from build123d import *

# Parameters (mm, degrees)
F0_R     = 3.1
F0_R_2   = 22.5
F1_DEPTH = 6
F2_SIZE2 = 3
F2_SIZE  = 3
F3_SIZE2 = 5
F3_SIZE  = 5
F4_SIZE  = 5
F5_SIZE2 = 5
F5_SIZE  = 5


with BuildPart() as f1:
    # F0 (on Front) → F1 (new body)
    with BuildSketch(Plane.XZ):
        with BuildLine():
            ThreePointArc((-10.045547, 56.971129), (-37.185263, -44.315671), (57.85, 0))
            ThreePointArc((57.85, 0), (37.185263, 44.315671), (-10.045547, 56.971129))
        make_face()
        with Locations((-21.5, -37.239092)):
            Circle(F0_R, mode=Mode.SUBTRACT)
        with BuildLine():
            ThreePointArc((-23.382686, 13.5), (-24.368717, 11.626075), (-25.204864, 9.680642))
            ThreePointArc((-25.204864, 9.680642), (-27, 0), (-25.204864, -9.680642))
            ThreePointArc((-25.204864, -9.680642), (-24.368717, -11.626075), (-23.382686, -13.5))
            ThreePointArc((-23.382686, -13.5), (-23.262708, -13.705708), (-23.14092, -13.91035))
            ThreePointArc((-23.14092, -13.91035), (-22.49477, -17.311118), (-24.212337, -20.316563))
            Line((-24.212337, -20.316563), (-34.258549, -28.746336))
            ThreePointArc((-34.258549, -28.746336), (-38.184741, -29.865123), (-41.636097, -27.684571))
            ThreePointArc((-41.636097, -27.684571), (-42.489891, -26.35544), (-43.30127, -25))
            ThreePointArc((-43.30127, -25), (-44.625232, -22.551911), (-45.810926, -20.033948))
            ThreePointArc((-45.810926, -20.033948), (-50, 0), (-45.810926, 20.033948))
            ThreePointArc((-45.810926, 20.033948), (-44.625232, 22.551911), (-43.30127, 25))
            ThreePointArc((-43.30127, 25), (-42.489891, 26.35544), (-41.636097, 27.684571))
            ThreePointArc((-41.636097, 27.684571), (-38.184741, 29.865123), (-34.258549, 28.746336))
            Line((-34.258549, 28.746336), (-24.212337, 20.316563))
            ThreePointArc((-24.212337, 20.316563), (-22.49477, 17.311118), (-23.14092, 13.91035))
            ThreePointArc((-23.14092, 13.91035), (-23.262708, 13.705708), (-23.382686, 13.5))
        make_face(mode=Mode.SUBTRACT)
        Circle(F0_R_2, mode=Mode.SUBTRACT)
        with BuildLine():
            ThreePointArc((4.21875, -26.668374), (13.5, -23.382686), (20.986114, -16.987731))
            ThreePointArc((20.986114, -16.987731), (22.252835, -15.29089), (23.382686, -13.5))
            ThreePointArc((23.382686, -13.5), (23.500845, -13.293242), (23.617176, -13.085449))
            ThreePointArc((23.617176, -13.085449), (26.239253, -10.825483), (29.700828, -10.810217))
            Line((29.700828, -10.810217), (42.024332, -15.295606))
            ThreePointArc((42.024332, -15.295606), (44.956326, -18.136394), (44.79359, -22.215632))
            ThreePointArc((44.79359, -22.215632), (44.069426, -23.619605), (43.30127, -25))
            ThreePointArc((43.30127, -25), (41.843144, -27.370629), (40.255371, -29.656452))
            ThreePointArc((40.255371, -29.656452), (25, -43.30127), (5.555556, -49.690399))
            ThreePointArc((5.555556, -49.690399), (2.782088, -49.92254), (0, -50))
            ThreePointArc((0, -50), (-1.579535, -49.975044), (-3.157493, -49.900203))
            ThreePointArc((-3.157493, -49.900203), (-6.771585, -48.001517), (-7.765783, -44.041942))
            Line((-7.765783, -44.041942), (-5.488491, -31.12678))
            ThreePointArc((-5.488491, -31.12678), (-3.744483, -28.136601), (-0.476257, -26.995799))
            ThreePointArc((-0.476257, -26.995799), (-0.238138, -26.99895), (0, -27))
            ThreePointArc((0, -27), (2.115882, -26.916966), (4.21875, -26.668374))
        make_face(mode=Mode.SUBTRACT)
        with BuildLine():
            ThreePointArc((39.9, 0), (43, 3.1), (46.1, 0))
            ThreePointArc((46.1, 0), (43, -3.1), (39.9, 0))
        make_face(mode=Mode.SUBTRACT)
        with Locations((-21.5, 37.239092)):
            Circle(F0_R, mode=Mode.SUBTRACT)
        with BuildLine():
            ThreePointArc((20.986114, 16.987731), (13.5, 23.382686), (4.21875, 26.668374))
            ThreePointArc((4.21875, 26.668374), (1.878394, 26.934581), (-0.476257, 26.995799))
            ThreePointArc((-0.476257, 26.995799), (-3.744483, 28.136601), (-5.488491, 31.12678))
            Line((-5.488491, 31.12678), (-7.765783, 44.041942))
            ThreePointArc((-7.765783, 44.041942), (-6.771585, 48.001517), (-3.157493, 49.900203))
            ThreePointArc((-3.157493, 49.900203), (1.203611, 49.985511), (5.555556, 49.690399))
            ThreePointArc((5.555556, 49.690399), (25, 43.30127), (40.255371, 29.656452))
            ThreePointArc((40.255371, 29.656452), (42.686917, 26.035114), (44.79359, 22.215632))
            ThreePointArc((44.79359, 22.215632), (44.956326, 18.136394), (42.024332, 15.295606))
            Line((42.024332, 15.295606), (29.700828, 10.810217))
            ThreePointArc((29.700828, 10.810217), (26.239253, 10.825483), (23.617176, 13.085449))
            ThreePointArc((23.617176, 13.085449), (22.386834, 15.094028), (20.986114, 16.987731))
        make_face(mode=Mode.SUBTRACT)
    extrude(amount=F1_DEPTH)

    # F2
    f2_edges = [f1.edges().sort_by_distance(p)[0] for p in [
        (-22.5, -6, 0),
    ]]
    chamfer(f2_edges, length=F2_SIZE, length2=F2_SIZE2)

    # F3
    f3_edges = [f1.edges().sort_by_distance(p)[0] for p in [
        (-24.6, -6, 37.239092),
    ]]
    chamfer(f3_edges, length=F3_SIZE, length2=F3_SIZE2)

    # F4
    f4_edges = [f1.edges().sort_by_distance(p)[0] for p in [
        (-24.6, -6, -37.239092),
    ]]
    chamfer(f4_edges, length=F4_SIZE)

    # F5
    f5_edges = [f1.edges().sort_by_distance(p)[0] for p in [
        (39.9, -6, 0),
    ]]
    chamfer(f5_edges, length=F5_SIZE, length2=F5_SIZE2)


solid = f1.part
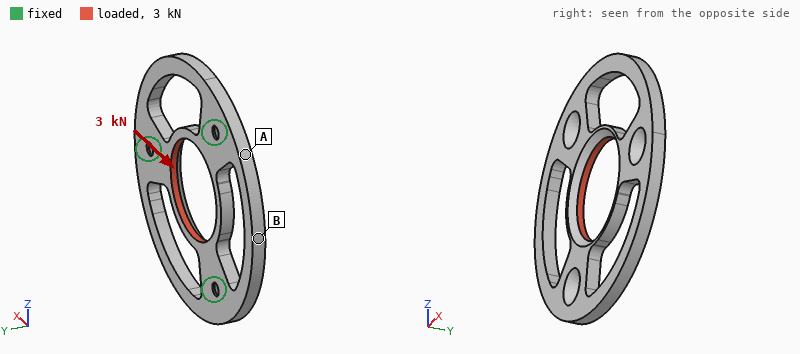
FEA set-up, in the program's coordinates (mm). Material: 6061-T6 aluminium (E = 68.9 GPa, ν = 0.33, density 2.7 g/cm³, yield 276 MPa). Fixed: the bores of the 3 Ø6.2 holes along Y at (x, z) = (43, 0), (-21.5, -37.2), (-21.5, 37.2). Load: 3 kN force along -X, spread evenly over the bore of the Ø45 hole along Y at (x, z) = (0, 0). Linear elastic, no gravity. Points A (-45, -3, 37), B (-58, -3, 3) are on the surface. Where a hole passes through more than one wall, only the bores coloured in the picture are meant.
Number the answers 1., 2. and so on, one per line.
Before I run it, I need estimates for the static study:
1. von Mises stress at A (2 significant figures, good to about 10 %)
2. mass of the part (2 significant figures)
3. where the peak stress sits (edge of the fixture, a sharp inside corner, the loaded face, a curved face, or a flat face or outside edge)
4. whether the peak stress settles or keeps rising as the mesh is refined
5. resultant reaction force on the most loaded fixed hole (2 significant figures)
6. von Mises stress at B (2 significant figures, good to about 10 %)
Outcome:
1. 29 MPa
2. 79 g
3. edge of the fixture
4. keeps rising
5. 1.3 kN
6. 10 MPa
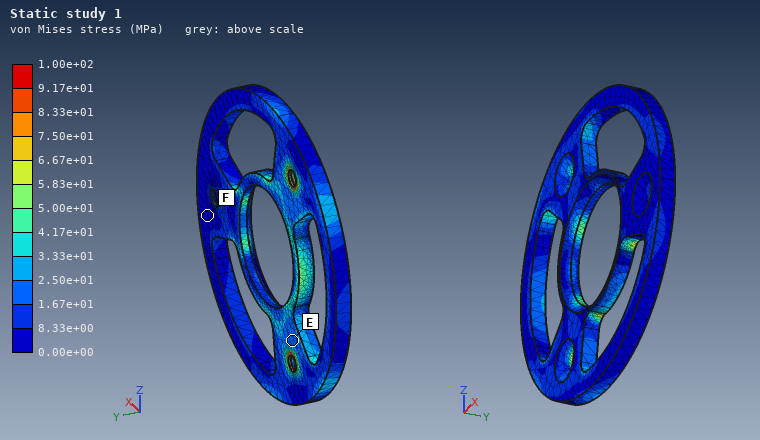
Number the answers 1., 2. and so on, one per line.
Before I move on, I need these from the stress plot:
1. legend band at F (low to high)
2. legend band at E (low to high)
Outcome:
1. 0.00e+00 to 8.33e+00 MPa
2. 1.67e+01 to 2.50e+01 MPa
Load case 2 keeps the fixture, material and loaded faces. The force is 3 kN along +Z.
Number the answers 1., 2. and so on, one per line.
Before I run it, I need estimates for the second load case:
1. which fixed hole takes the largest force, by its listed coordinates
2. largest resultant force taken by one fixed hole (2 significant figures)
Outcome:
1. (43, 0)
2. 1.5 kN
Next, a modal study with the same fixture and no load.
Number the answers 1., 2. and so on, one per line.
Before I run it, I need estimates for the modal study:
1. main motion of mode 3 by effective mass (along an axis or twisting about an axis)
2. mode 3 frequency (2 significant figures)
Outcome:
1. along Y
2. 2700 Hz
